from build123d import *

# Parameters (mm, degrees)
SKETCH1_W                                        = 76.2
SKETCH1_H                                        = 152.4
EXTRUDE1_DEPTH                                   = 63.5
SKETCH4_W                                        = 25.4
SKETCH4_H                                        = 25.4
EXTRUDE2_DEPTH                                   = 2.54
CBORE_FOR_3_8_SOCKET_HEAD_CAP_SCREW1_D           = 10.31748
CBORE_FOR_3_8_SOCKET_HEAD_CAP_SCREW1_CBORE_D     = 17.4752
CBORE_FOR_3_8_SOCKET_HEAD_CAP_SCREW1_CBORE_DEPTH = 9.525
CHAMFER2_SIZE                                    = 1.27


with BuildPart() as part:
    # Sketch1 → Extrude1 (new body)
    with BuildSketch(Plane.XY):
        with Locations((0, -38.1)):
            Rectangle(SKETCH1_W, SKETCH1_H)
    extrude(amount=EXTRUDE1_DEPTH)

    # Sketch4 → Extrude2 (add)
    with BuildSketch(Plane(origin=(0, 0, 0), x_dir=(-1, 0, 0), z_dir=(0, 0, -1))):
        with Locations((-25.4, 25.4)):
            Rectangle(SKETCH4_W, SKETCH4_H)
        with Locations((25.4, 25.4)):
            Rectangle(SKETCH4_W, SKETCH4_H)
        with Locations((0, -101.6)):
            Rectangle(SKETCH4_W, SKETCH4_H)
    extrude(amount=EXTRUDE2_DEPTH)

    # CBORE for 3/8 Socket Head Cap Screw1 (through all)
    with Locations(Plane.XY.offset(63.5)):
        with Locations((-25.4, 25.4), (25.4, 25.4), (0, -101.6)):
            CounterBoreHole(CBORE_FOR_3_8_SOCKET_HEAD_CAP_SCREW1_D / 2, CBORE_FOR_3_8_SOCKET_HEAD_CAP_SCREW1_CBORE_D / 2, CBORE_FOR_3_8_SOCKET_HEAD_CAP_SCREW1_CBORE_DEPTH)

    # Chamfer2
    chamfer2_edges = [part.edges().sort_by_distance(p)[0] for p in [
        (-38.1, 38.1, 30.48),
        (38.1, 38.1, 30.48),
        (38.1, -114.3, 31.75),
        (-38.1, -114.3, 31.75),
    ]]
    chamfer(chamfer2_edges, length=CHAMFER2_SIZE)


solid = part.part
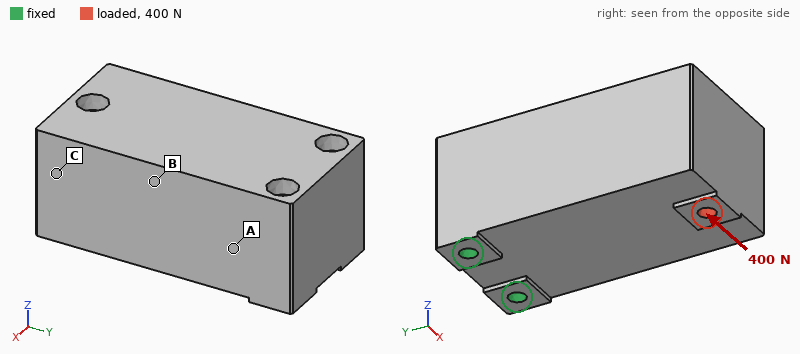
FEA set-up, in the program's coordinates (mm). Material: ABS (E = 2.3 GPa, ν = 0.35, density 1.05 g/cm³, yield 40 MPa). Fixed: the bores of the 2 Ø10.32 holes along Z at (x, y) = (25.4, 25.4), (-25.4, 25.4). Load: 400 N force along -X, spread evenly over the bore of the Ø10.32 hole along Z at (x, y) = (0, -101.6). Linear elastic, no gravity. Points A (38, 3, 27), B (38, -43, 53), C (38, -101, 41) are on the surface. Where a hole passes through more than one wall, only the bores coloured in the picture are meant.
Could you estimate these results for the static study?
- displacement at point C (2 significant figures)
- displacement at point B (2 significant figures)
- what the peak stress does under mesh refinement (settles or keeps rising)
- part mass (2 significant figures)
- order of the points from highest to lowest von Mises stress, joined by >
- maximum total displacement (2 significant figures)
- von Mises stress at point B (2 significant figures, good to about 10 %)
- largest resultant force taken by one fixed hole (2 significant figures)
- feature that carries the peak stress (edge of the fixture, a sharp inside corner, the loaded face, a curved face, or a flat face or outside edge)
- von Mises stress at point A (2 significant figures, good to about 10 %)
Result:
70 µm
33 µm
keeps rising
760 g
A > B > C
83 µm
0.37 MPa
930 N
edge of the fixture
0.65 MPa
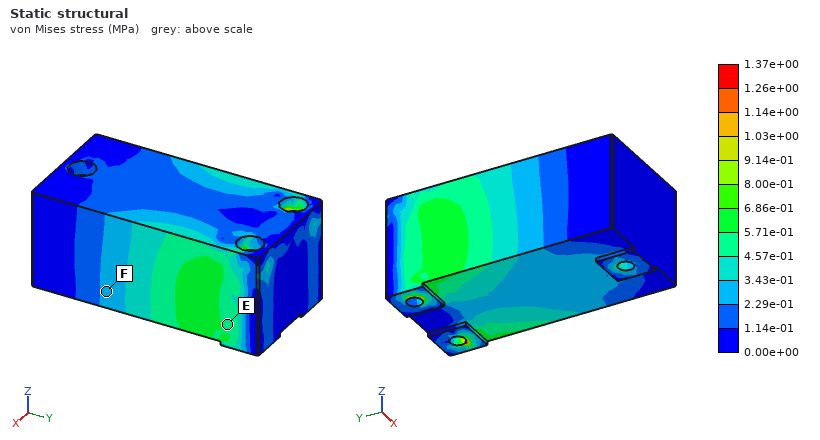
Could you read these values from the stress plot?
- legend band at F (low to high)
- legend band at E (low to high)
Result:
2.29e-01 to 3.43e-01 MPa
4.57e-01 to 5.71e-01 MPa
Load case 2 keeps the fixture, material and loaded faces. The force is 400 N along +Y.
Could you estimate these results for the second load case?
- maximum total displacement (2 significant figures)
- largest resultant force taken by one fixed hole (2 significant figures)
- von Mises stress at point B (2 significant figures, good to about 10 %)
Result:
11 µm
200 N
0.047 MPa
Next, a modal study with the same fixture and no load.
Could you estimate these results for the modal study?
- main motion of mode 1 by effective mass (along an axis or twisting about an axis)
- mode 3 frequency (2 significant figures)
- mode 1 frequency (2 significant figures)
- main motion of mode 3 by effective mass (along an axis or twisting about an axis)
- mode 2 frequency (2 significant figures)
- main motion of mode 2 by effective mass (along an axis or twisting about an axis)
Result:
along Z
1500 Hz
600 Hz
twisting about Y
770 Hz
along X
